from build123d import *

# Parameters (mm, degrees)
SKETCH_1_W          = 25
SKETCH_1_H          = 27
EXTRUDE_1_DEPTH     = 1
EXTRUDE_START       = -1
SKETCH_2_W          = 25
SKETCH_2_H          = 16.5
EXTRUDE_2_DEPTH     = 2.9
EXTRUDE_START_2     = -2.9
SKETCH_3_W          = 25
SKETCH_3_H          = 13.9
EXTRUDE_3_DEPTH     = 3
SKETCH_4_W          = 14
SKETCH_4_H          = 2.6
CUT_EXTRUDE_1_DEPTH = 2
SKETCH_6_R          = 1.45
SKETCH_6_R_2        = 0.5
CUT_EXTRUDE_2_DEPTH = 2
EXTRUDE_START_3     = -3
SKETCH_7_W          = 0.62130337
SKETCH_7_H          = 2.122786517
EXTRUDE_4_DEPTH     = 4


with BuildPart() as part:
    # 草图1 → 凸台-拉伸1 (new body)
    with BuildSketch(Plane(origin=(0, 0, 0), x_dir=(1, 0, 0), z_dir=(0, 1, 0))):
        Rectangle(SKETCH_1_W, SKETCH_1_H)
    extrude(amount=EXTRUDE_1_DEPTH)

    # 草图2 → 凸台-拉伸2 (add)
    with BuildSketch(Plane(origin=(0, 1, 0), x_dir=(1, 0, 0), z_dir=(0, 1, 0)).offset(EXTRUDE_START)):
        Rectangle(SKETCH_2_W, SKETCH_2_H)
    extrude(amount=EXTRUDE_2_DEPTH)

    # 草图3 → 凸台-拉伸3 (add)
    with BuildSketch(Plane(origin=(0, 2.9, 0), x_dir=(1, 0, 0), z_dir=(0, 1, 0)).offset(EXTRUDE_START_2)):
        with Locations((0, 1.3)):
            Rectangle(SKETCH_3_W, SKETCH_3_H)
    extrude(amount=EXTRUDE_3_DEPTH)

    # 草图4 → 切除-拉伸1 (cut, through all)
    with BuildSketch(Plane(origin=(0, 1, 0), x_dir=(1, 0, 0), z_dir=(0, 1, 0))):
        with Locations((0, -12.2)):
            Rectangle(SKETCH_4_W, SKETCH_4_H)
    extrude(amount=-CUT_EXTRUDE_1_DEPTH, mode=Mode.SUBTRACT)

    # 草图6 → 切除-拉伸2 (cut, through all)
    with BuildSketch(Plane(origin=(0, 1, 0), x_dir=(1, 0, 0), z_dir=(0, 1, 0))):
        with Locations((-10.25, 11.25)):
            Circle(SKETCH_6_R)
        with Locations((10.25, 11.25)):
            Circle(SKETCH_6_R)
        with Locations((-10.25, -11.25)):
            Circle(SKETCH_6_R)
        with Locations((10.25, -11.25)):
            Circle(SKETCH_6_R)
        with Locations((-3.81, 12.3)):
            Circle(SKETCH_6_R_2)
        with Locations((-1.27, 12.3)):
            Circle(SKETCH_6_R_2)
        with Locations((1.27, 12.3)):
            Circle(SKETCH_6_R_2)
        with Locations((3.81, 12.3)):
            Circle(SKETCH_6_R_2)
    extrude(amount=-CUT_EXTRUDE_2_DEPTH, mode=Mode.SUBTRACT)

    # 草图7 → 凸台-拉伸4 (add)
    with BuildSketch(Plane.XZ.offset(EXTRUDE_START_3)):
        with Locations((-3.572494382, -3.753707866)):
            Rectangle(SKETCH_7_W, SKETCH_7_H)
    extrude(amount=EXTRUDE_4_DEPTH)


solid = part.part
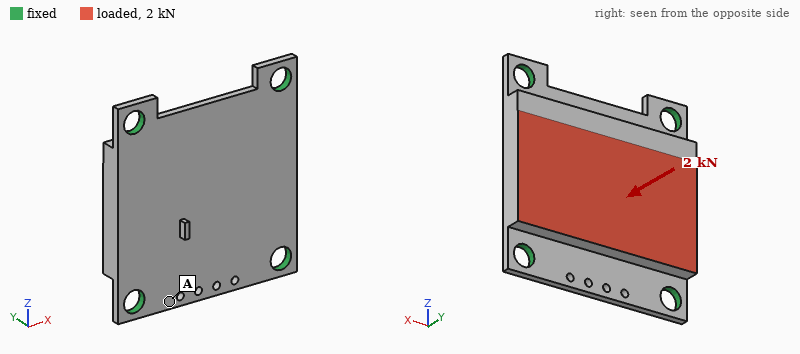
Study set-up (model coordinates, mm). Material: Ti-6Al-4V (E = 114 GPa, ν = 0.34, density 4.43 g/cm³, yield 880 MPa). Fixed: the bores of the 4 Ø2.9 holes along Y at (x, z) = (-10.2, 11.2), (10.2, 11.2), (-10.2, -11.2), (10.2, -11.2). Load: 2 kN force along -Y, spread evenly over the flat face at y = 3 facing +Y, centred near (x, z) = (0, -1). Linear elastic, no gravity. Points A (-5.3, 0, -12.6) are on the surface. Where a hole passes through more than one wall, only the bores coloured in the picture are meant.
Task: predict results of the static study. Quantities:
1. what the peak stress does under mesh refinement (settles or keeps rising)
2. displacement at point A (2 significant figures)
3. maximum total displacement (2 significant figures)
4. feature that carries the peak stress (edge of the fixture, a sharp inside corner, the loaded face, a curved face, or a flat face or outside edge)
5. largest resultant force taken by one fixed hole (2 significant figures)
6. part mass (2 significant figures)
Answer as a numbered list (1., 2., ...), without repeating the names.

1. keeps rising
2. 15 µm
3. 51 µm
4. edge of the fixture
5. 870 N
6. 6.3 g
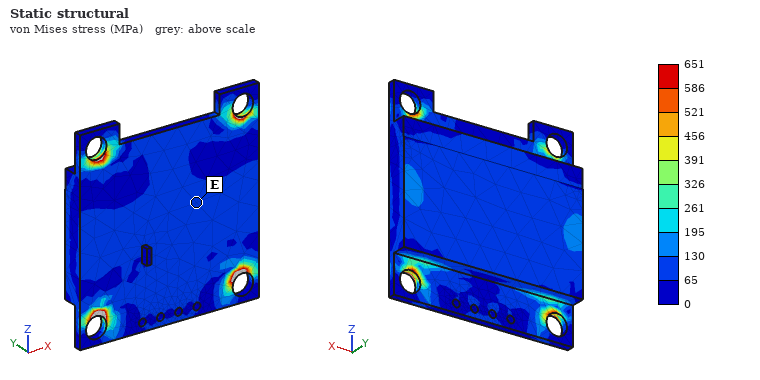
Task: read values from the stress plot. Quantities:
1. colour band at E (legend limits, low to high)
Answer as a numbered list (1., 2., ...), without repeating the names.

1. 65 to 130 MPa
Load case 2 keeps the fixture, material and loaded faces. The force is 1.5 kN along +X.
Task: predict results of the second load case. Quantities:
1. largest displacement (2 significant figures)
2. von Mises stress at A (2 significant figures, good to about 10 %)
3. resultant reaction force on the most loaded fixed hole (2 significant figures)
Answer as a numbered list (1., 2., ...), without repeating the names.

1. 11 µm
2. 20 MPa
3. 490 N
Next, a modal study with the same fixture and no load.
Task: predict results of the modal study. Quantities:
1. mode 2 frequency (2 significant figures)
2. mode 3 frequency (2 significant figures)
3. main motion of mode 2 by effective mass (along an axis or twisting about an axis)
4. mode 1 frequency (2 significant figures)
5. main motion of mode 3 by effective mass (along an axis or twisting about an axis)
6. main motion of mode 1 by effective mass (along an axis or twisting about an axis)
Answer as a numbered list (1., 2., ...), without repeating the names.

1. 23 kHz
2. 25 kHz
3. twisting about Z
4. 15 kHz
5. twisting about X
6. along Y
